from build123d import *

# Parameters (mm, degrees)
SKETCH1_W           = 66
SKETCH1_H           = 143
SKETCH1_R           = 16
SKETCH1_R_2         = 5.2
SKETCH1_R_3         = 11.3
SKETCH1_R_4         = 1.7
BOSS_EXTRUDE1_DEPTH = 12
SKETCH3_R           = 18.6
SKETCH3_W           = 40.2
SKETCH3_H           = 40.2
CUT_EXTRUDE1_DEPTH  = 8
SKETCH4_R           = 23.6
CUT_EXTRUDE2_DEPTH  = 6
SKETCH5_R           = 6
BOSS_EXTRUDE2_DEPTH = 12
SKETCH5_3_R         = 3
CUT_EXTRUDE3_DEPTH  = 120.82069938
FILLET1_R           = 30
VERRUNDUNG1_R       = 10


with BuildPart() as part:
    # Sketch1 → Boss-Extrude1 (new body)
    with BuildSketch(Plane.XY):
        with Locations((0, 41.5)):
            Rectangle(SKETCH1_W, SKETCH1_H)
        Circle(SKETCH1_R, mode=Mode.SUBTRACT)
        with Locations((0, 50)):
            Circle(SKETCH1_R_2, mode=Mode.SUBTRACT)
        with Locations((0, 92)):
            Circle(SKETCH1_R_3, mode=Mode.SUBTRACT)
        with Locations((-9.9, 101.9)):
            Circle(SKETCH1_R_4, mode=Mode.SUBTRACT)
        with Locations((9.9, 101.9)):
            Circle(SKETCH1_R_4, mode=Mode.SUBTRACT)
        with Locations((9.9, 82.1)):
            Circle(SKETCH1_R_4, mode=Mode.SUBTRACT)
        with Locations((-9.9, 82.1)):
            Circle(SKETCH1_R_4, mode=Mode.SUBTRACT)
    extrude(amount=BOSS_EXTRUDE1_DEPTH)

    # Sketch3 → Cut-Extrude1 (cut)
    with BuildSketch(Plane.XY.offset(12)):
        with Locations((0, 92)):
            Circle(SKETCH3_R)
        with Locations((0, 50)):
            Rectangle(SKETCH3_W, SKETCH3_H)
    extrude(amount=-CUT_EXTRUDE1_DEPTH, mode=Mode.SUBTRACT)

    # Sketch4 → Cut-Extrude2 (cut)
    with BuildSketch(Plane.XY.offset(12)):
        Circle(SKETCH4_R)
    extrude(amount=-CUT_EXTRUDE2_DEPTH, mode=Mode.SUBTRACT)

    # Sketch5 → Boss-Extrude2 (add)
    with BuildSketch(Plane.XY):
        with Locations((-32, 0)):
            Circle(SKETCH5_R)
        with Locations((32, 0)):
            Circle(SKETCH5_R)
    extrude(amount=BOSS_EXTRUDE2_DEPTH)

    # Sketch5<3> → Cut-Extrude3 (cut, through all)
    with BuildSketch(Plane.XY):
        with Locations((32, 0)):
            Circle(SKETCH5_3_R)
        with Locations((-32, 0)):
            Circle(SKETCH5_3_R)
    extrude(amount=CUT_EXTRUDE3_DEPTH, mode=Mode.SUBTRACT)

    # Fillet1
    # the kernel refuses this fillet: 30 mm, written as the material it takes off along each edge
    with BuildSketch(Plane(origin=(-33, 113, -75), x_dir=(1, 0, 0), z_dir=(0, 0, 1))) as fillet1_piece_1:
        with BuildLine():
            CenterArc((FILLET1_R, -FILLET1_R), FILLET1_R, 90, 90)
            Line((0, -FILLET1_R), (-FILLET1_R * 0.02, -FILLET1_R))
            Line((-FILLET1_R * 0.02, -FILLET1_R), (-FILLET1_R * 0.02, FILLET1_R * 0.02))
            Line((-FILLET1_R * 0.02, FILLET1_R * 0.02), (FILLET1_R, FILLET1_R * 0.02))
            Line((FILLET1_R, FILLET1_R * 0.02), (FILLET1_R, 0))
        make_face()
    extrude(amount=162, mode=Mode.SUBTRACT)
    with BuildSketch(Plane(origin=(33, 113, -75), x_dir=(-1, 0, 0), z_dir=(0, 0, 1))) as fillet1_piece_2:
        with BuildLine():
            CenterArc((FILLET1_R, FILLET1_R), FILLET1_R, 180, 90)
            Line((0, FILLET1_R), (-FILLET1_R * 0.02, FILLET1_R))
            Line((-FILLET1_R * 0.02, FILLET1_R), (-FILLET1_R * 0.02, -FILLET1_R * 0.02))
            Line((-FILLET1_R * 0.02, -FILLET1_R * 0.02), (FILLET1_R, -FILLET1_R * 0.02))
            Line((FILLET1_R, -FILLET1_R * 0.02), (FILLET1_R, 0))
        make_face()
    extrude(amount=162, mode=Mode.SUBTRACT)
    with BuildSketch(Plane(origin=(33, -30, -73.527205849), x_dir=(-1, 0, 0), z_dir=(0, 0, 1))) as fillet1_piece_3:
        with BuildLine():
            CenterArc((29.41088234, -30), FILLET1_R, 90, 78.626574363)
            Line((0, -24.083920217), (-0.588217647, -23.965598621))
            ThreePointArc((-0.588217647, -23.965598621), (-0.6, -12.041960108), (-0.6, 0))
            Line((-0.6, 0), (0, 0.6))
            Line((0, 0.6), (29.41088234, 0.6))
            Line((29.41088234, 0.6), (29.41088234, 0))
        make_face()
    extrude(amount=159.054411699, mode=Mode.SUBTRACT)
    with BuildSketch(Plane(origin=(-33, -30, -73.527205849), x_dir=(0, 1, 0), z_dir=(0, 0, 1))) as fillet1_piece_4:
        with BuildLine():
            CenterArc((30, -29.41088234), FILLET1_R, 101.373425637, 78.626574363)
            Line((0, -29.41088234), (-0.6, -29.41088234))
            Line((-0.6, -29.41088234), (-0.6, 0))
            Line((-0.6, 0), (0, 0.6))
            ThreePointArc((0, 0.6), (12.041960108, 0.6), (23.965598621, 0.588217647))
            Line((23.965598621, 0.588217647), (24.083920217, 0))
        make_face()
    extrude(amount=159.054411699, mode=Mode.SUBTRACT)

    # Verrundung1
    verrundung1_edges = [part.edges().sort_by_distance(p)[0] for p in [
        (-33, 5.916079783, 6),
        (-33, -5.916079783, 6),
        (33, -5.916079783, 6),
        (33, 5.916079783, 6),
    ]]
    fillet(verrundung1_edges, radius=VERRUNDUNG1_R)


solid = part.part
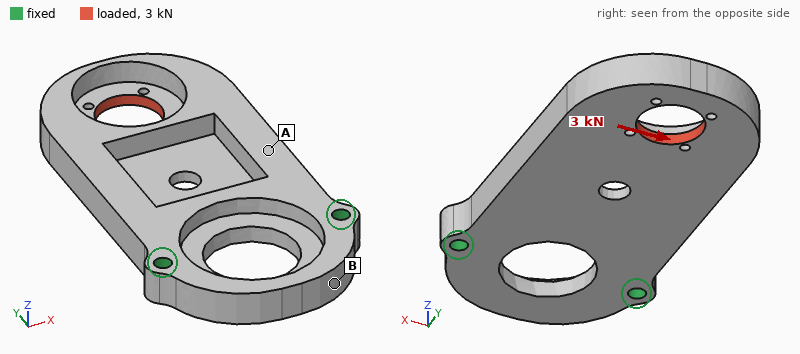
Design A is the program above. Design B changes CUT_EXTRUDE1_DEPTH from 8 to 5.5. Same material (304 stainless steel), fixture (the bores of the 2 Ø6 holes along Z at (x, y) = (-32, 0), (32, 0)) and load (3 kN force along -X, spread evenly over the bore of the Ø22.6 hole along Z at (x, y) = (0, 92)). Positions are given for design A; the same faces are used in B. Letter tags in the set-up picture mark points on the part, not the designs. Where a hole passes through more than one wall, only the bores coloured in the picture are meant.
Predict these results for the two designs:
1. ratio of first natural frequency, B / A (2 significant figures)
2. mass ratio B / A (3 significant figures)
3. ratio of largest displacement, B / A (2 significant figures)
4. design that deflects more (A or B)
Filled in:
0.95
1.08
0.81
A
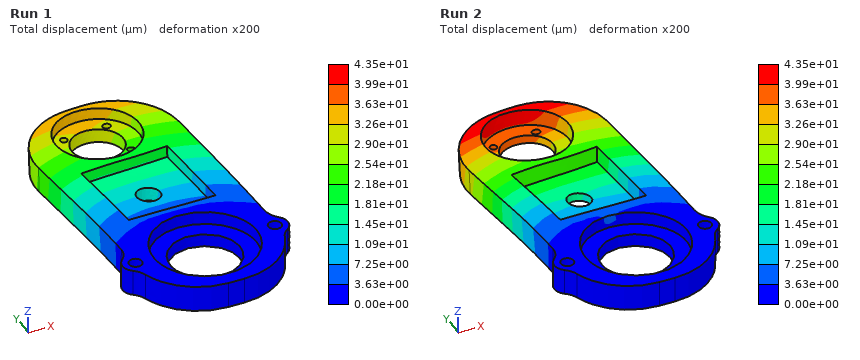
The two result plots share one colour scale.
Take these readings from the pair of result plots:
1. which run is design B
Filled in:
Run 1
